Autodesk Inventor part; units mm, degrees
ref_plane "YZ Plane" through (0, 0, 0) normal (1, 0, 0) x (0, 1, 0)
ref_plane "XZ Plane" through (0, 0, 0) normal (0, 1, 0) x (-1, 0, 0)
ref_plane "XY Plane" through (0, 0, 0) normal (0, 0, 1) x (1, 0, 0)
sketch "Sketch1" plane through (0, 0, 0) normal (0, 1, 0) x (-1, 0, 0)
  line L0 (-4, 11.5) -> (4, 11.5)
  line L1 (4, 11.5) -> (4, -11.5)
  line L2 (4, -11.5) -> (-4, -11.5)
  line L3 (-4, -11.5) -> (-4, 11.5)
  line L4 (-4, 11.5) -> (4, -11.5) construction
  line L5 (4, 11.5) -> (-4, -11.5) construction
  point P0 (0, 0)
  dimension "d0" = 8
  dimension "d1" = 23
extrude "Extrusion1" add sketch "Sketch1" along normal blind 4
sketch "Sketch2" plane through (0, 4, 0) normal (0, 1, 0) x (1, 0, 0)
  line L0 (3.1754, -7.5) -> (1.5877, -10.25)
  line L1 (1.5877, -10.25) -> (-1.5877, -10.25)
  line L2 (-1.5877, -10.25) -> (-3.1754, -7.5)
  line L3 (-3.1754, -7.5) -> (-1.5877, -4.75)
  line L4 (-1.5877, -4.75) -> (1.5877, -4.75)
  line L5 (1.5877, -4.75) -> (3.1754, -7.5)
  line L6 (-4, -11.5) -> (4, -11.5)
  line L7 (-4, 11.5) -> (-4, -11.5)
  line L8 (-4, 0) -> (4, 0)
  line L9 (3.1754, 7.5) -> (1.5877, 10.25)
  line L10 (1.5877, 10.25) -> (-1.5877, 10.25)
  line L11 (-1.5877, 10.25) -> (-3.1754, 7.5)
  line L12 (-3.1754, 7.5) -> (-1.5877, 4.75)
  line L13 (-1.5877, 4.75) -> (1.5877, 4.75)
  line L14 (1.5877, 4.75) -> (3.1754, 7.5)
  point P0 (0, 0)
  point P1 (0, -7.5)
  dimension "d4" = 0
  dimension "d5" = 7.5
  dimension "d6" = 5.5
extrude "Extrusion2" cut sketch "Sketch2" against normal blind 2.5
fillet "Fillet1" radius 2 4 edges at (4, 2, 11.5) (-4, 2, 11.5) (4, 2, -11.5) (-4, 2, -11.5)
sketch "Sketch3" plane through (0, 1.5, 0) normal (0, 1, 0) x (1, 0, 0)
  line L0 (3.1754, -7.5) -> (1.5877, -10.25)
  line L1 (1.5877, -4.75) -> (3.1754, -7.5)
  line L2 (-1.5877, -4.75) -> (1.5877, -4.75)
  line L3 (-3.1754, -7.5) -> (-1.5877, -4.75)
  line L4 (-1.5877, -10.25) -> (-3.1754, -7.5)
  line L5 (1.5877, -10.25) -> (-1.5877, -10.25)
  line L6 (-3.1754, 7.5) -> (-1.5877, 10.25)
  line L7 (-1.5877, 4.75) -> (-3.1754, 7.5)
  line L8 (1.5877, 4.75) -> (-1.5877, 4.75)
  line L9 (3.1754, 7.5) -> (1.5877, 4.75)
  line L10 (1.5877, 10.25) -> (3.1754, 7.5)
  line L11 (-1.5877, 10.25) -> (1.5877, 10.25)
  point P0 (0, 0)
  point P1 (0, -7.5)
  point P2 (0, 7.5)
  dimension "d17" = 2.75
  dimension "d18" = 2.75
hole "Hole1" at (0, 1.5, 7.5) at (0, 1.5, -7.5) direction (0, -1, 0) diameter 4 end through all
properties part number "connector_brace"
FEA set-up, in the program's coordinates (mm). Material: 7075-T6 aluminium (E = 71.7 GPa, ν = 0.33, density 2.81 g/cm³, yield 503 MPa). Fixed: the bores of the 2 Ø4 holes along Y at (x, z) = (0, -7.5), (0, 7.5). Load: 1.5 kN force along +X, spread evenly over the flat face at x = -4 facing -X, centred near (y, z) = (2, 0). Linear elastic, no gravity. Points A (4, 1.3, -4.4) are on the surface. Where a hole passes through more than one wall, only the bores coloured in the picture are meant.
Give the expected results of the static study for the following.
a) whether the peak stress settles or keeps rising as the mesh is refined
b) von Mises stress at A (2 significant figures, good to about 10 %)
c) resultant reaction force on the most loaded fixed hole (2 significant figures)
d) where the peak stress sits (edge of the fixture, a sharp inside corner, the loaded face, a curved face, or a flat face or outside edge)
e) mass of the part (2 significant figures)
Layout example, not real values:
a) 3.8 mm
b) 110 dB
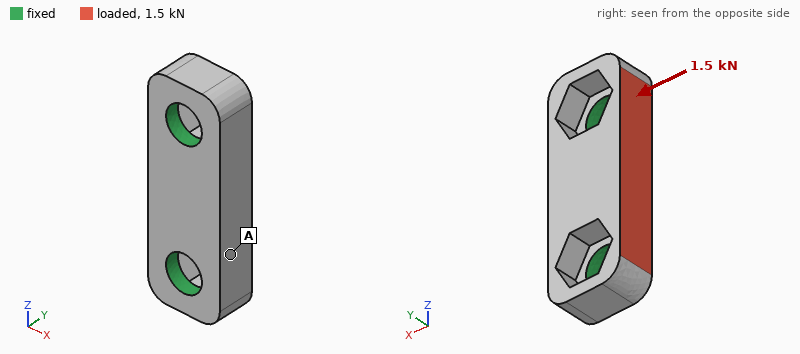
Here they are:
a) keeps rising
b) 18 MPa
c) 750 N
d) edge of the fixture
e) 1.6 g
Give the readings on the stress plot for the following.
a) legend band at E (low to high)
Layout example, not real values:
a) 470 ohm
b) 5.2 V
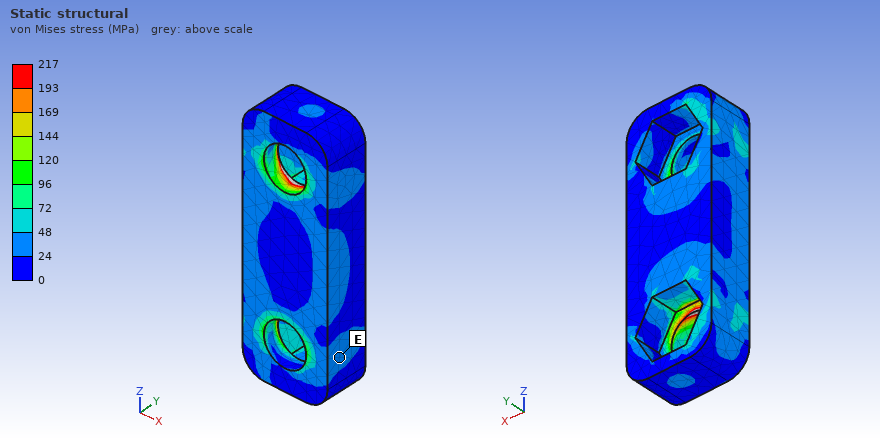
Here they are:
a) 24 to 48 MPa
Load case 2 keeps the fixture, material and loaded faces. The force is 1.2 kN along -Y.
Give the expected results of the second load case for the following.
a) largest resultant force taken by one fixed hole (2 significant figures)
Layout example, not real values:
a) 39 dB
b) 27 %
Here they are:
a) 640 N
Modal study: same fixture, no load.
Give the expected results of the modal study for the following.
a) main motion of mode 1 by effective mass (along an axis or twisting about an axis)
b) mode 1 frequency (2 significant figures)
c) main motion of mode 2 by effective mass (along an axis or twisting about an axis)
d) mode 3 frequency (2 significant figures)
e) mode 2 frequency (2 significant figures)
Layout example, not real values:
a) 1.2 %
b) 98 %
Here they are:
a) along X
b) 49 kHz
c) along Y
d) 84 kHz
e) 61 kHz
